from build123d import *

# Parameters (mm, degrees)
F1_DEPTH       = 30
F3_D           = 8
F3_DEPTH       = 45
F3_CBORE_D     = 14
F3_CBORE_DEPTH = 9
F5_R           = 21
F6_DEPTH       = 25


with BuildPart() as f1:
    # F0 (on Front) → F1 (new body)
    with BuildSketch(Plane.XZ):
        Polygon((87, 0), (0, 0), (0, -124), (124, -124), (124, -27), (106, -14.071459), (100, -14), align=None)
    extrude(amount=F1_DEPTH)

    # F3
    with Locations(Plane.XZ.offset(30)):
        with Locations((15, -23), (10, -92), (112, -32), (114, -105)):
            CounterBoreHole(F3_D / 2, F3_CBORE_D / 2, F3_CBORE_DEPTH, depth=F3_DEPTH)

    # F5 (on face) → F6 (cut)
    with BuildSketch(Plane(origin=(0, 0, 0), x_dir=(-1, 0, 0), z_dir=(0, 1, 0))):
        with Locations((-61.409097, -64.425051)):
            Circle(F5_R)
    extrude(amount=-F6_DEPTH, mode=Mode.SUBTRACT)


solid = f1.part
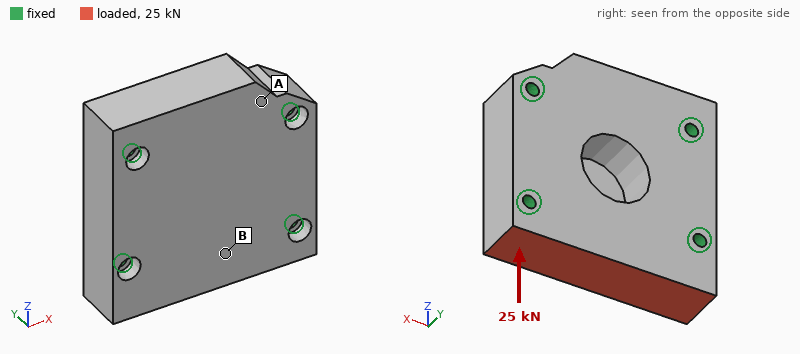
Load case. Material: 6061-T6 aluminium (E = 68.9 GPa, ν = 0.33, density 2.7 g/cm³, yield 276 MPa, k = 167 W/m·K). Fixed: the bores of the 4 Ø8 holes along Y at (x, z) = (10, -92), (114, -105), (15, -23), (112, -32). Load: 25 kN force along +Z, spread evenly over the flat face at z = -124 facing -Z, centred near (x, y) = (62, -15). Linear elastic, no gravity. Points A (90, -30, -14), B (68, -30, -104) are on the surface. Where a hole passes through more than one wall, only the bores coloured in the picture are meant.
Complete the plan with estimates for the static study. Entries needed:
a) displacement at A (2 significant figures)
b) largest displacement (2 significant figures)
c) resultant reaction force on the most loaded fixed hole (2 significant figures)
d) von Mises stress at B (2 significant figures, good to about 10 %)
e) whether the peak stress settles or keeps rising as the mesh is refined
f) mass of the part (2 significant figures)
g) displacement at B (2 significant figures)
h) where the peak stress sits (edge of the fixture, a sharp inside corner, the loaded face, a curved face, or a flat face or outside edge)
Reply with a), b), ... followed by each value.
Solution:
a) 2.6 µm
b) 11 µm
c) 8.9 kN
d) 5.9 MPa
e) keeps rising
f) 1.1 kg
g) 9.3 µm
h) edge of the fixture
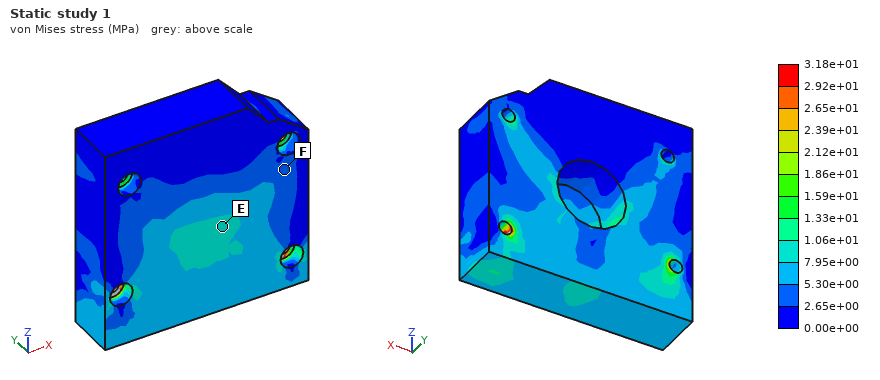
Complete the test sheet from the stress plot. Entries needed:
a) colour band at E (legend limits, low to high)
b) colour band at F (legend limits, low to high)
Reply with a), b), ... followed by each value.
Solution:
a) 7.95e+00 to 1.06e+01 MPa
b) 2.65e+00 to 5.30e+00 MPa
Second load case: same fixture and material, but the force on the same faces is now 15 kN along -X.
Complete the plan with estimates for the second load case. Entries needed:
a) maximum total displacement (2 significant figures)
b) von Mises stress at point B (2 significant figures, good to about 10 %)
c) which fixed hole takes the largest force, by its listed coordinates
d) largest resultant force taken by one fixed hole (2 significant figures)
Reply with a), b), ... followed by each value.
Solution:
a) 12 µm
b) 5.2 MPa
c) (114, -105)
d) 8.4 kN
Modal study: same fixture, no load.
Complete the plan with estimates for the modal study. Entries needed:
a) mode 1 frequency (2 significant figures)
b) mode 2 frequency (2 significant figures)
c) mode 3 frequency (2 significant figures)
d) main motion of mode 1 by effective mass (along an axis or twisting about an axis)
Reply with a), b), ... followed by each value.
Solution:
a) 7300 Hz
b) 8200 Hz
c) 11 kHz
d) along Y
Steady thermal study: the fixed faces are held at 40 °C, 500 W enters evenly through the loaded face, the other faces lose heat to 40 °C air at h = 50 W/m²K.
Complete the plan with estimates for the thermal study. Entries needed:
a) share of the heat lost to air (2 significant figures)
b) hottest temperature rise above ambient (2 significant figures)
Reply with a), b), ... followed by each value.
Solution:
a) 4.4 %
b) 42 K
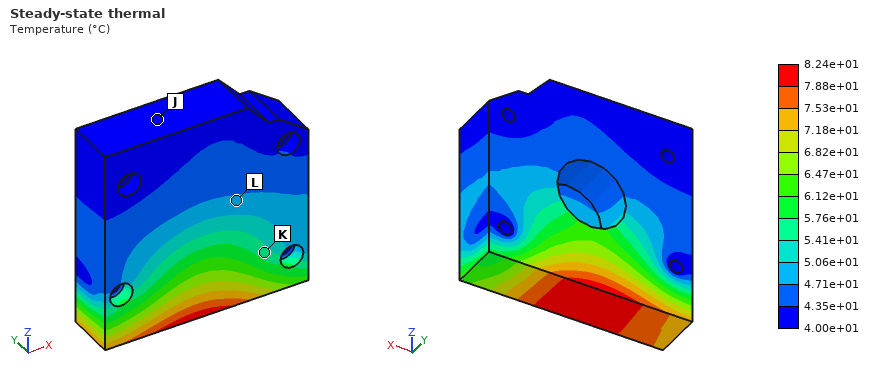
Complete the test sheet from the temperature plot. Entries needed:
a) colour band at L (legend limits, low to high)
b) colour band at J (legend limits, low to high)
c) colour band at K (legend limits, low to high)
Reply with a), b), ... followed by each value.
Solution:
a) 4.71e+01 to 5.06e+01 °C
b) 4.00e+01 to 4.35e+01 °C
c) 5.41e+01 to 5.76e+01 °C
